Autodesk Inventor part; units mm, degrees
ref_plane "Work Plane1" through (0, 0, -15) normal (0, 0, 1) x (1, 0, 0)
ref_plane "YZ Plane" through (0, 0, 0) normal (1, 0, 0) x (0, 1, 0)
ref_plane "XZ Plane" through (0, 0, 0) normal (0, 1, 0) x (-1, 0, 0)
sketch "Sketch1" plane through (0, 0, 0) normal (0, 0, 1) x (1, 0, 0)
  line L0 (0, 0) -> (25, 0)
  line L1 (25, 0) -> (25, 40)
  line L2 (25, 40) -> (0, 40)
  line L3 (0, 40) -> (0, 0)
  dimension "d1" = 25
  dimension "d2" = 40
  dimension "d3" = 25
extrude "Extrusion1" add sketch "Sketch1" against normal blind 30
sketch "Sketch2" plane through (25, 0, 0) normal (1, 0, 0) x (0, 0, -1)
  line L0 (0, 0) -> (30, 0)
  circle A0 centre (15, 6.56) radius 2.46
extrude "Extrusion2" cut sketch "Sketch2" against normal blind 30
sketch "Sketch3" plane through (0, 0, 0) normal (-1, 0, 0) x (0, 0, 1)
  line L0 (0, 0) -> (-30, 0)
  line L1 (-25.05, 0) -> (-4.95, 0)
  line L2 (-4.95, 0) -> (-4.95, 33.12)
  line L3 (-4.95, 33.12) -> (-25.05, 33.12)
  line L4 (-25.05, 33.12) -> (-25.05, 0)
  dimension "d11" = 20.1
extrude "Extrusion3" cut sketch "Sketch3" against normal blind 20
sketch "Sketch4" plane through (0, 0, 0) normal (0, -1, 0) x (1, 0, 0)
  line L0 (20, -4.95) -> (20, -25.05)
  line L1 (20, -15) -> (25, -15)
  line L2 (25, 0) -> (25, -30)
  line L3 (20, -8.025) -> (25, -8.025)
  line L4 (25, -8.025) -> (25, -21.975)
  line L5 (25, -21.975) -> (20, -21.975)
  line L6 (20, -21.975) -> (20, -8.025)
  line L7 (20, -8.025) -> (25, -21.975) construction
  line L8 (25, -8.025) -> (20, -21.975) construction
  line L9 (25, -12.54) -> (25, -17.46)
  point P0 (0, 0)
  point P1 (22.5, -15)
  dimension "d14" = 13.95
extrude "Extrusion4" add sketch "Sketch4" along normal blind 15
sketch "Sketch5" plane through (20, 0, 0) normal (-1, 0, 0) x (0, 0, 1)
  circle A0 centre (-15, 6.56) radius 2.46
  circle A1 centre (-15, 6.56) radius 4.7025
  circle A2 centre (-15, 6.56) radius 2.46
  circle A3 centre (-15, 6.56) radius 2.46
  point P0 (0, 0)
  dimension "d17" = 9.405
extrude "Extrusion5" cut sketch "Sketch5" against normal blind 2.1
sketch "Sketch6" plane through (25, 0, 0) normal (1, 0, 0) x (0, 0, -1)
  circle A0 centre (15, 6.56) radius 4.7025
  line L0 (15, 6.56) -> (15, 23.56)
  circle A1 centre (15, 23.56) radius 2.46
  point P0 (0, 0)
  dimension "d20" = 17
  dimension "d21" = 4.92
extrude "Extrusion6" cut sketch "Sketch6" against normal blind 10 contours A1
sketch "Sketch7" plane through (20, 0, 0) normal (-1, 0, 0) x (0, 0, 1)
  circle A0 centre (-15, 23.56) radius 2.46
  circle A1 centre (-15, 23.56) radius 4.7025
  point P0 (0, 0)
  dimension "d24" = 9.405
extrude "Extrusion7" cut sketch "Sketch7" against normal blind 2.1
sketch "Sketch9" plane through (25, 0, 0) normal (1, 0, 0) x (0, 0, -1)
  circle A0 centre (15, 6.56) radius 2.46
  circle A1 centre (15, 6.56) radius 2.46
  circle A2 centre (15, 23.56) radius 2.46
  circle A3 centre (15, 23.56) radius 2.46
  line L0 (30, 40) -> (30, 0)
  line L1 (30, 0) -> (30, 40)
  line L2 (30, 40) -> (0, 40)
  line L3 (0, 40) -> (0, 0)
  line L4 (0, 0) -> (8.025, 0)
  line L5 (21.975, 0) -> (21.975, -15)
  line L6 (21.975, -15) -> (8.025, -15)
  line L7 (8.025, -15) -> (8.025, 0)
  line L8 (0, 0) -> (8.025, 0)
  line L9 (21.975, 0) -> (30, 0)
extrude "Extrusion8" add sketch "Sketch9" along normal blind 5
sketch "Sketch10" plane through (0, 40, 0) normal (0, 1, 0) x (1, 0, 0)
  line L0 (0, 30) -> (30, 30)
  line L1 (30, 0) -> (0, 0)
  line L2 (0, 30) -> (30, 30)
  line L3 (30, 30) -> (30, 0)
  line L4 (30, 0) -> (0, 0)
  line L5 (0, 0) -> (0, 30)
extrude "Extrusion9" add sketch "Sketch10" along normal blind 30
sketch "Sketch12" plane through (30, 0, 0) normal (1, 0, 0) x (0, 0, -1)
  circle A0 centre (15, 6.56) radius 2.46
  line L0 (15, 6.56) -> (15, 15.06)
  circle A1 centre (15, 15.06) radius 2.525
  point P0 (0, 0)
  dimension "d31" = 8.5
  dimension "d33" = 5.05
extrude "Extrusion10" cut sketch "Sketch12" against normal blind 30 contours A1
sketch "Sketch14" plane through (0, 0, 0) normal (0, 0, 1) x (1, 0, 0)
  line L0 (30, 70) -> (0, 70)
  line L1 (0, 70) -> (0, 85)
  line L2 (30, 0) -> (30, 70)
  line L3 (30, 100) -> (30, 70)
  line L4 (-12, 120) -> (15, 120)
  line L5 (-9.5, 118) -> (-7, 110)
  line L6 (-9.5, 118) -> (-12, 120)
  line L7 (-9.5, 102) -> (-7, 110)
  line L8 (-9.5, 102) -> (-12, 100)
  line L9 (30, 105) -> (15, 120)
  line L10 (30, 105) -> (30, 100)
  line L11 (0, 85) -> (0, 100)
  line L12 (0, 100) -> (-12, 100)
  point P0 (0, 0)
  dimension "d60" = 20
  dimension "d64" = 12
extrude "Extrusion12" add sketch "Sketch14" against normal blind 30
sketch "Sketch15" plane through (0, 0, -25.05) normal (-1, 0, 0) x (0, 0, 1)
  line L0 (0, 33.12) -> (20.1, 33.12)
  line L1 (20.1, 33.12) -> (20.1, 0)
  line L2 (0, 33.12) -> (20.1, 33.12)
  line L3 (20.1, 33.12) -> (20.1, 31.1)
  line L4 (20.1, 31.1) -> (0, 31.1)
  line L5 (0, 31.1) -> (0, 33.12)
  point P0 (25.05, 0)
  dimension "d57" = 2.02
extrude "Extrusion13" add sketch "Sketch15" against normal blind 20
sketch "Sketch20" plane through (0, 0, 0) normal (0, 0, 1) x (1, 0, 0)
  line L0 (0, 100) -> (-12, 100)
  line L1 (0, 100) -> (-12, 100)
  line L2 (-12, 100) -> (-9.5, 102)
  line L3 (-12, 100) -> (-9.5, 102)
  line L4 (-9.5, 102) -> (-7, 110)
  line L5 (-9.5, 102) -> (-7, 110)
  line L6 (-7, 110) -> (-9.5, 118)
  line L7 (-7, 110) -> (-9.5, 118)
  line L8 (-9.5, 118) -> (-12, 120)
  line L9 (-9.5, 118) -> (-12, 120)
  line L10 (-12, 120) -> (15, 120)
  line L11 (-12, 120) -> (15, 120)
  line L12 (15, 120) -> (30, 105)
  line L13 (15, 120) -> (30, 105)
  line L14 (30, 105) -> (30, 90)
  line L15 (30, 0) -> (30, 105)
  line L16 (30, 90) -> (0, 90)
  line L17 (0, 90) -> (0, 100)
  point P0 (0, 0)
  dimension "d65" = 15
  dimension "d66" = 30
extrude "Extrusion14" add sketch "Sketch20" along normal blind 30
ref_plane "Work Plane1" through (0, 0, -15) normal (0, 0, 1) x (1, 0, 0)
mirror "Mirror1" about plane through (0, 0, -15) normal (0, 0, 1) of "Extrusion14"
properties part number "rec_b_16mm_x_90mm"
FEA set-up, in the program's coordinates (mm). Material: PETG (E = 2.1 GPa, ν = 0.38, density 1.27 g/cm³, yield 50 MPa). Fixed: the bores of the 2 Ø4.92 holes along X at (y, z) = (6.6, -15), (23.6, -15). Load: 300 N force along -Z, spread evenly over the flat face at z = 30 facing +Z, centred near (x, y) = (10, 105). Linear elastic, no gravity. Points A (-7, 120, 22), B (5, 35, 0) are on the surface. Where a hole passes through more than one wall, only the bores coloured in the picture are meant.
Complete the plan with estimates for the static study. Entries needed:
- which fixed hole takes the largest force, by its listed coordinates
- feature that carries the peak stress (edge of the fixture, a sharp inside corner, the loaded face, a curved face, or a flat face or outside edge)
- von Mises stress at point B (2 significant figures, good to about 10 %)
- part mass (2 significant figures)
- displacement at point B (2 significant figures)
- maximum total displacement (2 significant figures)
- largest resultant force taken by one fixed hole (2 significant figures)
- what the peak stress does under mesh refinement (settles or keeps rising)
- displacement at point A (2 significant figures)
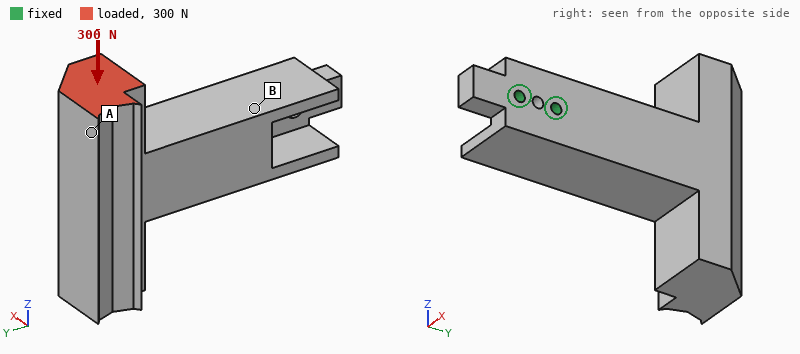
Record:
(23.6, -15)
edge of the fixture
4.7 MPa
200 g
0.29 mm
1.9 mm
1.4 kN
keeps rising
1.8 mm
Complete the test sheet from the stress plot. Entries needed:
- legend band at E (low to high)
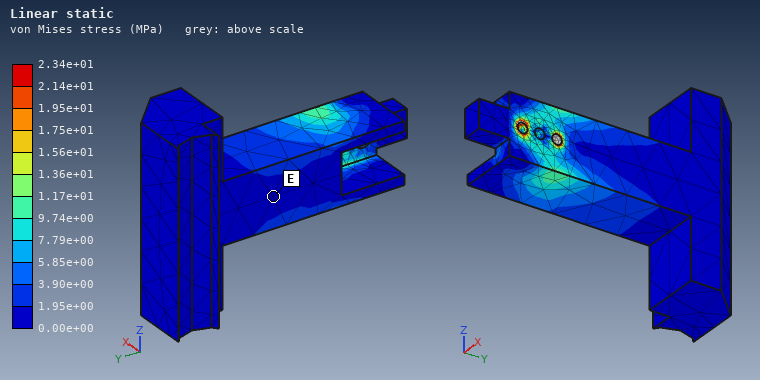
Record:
0.00e+00 to 1.95e+00 MPa
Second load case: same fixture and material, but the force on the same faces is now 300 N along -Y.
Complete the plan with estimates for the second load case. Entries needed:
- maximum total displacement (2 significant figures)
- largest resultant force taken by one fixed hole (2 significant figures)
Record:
1.4 mm
640 N
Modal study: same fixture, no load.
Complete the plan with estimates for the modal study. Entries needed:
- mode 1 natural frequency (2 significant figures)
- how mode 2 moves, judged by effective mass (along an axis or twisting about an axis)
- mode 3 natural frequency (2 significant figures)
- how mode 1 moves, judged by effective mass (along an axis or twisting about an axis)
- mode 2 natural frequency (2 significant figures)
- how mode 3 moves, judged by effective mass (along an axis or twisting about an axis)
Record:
180 Hz
along Z
340 Hz
along X
200 Hz
twisting about Y
